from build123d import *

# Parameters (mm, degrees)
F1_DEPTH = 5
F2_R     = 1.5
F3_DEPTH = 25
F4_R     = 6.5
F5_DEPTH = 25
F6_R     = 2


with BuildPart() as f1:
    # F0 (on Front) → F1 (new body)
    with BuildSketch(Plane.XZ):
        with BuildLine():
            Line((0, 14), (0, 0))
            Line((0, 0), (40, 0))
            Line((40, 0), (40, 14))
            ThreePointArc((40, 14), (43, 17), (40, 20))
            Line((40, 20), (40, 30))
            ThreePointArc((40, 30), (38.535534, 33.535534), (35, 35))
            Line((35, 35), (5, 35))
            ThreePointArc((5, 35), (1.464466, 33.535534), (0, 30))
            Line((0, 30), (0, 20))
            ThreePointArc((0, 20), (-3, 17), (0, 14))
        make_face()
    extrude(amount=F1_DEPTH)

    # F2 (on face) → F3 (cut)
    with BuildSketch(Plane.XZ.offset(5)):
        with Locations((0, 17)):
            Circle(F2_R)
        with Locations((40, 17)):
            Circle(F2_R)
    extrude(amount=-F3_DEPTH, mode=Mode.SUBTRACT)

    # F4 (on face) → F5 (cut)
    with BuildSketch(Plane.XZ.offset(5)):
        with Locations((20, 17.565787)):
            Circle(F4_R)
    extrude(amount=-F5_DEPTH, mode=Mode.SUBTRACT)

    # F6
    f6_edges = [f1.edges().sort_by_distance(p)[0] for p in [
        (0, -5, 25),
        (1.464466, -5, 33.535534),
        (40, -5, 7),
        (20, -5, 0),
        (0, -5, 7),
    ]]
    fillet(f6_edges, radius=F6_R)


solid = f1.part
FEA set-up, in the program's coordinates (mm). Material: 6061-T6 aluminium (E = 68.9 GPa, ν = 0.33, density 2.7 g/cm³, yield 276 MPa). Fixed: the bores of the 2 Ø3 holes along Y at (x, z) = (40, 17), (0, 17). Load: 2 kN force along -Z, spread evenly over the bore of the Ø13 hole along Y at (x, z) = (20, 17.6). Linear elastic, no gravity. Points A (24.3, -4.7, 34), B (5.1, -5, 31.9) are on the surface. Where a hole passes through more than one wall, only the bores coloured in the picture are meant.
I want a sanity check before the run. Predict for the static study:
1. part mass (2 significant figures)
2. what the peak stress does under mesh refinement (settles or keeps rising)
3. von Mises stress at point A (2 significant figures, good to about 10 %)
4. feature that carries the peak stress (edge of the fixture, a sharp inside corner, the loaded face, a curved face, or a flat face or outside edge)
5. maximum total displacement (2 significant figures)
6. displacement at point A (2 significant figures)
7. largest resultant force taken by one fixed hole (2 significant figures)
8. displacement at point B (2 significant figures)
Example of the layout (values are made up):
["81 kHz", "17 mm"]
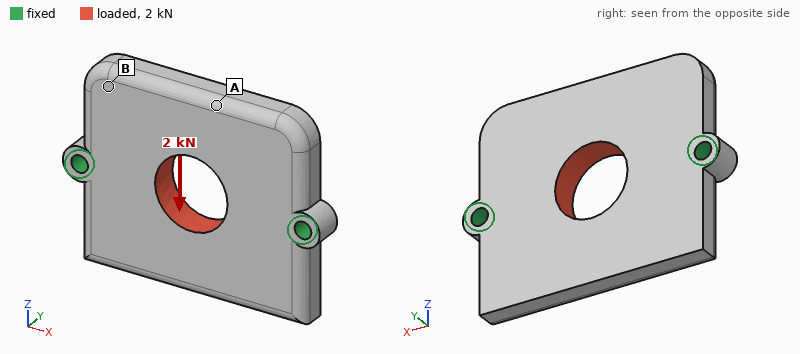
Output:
["17 g", "keeps rising", "15 MPa", "edge of the fixture", "7.9 µm", "6.5 µm", "1.0 kN", "4.2 µm"]
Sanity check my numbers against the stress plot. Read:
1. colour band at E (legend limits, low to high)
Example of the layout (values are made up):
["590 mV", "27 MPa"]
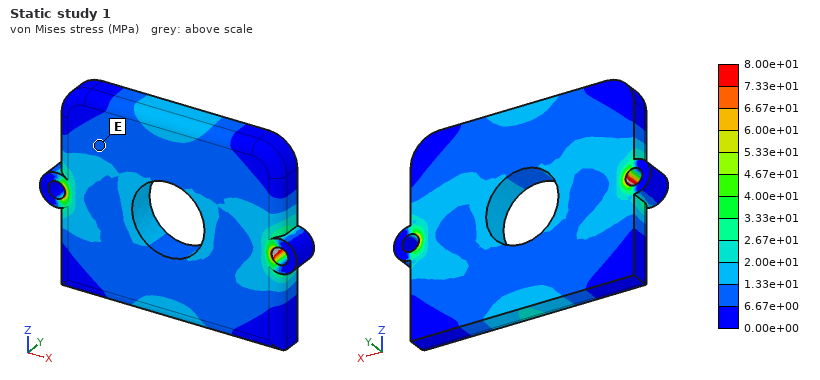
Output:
["6.67e+00 to 1.33e+01 MPa"]
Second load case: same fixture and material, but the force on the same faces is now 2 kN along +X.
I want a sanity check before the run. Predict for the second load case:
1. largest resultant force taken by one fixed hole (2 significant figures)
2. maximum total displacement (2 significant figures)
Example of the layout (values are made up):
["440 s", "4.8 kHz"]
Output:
["1.0 kN", "4.9 µm"]
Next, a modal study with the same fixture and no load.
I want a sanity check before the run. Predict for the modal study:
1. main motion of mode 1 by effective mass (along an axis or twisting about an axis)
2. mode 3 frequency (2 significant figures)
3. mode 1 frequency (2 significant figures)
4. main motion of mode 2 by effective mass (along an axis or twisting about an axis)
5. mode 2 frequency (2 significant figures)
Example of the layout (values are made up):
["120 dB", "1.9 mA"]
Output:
["twisting about X", "15 kHz", "6400 Hz", "along Y", "8800 Hz"]
